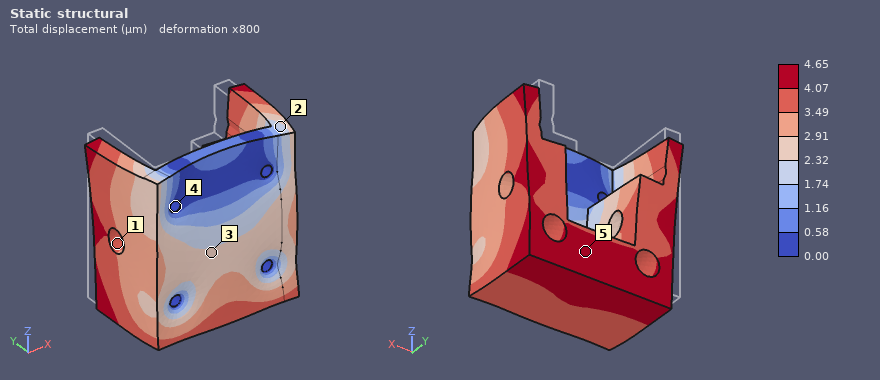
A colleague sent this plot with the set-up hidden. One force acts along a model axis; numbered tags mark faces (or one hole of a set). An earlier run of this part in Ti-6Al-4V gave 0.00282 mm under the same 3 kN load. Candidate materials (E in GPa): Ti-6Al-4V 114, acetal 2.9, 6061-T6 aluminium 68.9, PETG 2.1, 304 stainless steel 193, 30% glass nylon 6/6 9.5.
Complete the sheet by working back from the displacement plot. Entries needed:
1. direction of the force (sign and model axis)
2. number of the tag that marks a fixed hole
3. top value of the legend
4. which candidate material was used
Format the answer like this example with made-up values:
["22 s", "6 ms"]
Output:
["-Y", "4", "4.65 µm", "6061-T6 aluminium"]
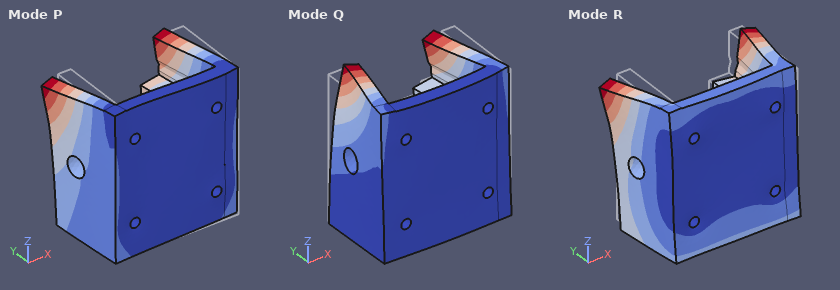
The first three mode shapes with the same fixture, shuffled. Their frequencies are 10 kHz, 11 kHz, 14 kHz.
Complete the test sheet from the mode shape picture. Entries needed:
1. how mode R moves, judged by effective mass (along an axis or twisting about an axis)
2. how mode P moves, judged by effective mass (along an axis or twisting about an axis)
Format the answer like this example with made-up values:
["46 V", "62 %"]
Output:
["along Z", "along X"]
